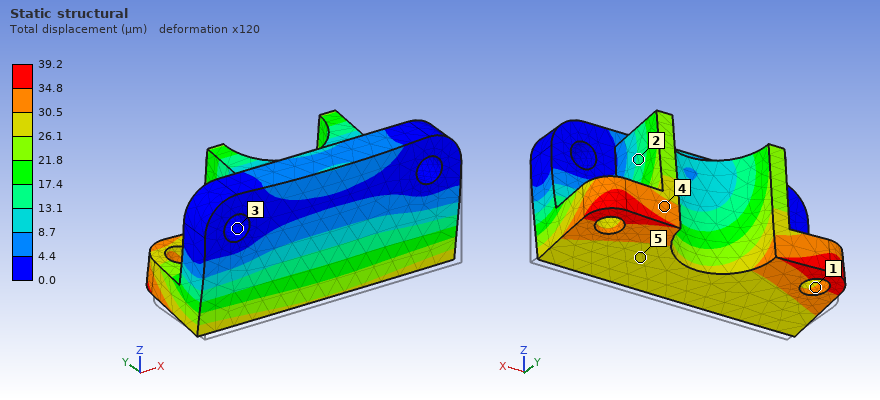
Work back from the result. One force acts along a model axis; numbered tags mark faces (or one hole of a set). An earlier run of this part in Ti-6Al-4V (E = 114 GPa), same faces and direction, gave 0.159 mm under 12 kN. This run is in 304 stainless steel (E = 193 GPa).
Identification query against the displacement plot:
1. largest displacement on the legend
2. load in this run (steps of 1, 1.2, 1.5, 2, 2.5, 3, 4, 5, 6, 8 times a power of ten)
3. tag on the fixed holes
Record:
39.2 µm
5 kN
3
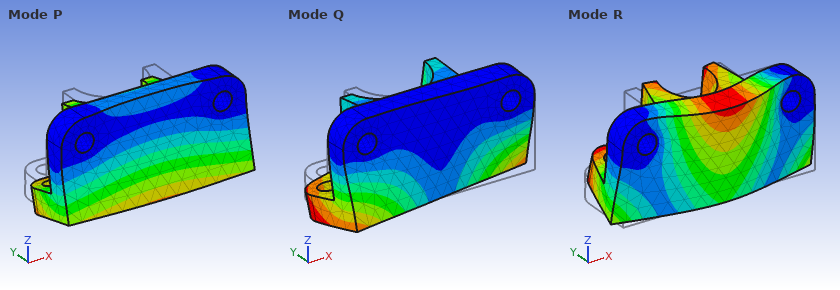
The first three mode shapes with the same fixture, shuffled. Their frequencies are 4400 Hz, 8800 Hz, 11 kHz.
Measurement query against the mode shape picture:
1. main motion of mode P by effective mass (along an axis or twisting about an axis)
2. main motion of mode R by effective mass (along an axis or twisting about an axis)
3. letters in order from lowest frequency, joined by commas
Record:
along Y
along Y
P, Q, R
